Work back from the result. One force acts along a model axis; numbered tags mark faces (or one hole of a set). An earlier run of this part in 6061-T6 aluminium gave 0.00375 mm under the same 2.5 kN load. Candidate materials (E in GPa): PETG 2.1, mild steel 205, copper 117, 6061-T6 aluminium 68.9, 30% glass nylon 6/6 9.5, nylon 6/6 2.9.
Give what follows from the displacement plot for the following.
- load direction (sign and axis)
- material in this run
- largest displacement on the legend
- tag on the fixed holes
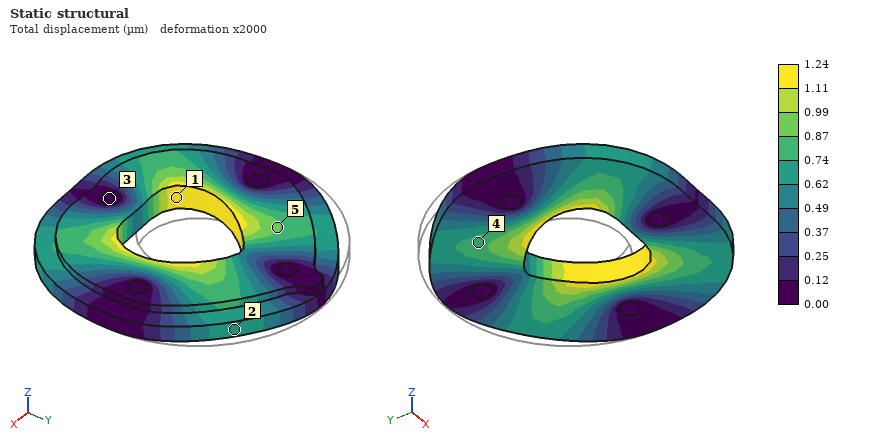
-Y
mild steel
1.24 µm
3
